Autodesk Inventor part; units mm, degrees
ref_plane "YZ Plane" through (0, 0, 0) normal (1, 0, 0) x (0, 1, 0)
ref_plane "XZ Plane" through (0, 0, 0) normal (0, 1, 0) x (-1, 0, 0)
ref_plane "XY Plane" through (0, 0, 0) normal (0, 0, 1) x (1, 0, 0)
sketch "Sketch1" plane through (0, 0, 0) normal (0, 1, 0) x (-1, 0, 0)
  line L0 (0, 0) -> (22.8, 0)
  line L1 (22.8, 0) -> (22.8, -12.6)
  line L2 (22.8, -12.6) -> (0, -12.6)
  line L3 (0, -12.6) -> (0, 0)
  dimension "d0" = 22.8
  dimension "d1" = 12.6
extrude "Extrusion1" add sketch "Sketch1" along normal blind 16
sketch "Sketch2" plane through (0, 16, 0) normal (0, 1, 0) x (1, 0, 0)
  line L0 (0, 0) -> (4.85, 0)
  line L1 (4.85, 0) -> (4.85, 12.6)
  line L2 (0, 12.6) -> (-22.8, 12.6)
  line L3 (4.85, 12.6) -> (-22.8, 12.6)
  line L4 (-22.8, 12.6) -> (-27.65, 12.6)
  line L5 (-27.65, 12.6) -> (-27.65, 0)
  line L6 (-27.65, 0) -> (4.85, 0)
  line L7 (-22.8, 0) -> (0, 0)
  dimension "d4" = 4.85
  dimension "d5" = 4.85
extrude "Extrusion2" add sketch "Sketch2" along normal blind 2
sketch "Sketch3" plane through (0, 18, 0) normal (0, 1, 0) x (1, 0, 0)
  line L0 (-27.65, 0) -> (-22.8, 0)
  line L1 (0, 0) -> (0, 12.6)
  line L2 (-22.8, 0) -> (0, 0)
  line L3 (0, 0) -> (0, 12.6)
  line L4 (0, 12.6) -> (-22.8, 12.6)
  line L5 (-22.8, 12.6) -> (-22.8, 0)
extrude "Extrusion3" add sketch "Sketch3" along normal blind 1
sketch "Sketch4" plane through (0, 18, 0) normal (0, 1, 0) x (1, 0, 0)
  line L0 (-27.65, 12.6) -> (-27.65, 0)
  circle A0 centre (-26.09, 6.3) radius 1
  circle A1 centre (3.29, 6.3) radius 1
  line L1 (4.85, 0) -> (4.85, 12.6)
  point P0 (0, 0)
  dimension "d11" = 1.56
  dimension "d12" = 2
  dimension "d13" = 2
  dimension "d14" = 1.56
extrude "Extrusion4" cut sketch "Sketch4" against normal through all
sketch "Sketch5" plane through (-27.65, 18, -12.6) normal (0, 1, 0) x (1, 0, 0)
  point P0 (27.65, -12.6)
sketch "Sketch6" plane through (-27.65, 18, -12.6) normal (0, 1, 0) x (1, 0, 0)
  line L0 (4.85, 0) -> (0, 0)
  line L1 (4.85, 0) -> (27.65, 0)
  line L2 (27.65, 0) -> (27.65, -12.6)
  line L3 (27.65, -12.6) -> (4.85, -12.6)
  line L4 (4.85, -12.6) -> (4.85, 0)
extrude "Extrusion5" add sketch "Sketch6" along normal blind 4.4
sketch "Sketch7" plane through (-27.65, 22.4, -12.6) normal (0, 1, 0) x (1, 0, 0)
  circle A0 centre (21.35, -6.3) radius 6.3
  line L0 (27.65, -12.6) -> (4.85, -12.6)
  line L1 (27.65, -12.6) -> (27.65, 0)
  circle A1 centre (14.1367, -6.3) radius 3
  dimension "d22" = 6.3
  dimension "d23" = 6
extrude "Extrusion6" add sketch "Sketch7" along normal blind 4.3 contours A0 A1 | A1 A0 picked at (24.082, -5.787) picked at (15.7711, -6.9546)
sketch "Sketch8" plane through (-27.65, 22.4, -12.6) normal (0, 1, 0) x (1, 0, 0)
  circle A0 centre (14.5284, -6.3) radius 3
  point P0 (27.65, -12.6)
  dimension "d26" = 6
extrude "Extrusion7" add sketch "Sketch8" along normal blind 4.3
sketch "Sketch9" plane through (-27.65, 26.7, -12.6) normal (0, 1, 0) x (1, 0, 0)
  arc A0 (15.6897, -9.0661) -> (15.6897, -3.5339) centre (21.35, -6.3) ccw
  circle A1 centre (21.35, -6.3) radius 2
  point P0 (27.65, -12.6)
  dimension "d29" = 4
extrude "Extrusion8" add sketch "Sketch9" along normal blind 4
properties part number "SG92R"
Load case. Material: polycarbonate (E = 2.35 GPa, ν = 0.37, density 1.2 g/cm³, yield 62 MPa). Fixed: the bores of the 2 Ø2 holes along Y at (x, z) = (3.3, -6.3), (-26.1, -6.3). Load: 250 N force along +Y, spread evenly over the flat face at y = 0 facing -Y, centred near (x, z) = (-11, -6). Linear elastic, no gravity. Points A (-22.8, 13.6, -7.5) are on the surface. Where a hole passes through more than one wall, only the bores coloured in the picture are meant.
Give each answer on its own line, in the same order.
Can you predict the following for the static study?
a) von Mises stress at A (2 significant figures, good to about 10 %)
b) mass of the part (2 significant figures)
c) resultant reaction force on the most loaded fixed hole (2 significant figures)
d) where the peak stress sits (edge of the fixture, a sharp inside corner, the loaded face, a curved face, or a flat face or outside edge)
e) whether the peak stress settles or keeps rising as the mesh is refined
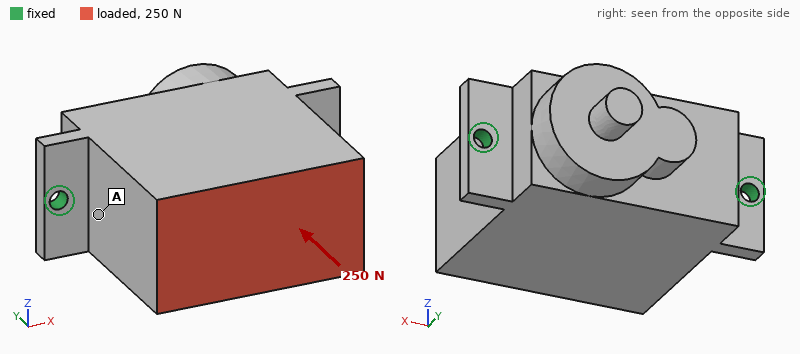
4.3 MPa
8.8 g
130 N
edge of the fixture
keeps rising
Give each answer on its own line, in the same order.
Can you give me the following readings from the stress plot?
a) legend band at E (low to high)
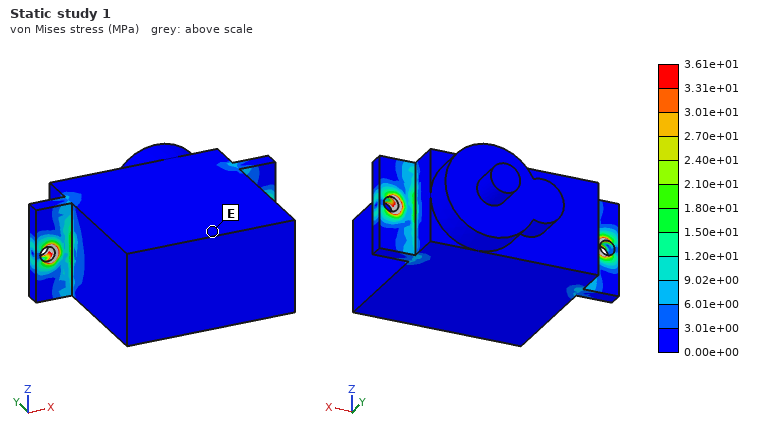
0.00e+00 to 3.01e+00 MPa
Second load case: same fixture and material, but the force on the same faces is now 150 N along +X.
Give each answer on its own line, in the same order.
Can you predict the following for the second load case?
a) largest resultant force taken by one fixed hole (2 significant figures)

120 N
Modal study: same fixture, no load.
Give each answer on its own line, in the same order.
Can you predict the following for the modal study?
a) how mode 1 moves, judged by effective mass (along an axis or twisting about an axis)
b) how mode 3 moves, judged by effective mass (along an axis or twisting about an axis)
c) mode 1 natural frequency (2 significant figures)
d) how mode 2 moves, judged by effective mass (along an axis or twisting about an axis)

along Z
along X
740 Hz
along Y
